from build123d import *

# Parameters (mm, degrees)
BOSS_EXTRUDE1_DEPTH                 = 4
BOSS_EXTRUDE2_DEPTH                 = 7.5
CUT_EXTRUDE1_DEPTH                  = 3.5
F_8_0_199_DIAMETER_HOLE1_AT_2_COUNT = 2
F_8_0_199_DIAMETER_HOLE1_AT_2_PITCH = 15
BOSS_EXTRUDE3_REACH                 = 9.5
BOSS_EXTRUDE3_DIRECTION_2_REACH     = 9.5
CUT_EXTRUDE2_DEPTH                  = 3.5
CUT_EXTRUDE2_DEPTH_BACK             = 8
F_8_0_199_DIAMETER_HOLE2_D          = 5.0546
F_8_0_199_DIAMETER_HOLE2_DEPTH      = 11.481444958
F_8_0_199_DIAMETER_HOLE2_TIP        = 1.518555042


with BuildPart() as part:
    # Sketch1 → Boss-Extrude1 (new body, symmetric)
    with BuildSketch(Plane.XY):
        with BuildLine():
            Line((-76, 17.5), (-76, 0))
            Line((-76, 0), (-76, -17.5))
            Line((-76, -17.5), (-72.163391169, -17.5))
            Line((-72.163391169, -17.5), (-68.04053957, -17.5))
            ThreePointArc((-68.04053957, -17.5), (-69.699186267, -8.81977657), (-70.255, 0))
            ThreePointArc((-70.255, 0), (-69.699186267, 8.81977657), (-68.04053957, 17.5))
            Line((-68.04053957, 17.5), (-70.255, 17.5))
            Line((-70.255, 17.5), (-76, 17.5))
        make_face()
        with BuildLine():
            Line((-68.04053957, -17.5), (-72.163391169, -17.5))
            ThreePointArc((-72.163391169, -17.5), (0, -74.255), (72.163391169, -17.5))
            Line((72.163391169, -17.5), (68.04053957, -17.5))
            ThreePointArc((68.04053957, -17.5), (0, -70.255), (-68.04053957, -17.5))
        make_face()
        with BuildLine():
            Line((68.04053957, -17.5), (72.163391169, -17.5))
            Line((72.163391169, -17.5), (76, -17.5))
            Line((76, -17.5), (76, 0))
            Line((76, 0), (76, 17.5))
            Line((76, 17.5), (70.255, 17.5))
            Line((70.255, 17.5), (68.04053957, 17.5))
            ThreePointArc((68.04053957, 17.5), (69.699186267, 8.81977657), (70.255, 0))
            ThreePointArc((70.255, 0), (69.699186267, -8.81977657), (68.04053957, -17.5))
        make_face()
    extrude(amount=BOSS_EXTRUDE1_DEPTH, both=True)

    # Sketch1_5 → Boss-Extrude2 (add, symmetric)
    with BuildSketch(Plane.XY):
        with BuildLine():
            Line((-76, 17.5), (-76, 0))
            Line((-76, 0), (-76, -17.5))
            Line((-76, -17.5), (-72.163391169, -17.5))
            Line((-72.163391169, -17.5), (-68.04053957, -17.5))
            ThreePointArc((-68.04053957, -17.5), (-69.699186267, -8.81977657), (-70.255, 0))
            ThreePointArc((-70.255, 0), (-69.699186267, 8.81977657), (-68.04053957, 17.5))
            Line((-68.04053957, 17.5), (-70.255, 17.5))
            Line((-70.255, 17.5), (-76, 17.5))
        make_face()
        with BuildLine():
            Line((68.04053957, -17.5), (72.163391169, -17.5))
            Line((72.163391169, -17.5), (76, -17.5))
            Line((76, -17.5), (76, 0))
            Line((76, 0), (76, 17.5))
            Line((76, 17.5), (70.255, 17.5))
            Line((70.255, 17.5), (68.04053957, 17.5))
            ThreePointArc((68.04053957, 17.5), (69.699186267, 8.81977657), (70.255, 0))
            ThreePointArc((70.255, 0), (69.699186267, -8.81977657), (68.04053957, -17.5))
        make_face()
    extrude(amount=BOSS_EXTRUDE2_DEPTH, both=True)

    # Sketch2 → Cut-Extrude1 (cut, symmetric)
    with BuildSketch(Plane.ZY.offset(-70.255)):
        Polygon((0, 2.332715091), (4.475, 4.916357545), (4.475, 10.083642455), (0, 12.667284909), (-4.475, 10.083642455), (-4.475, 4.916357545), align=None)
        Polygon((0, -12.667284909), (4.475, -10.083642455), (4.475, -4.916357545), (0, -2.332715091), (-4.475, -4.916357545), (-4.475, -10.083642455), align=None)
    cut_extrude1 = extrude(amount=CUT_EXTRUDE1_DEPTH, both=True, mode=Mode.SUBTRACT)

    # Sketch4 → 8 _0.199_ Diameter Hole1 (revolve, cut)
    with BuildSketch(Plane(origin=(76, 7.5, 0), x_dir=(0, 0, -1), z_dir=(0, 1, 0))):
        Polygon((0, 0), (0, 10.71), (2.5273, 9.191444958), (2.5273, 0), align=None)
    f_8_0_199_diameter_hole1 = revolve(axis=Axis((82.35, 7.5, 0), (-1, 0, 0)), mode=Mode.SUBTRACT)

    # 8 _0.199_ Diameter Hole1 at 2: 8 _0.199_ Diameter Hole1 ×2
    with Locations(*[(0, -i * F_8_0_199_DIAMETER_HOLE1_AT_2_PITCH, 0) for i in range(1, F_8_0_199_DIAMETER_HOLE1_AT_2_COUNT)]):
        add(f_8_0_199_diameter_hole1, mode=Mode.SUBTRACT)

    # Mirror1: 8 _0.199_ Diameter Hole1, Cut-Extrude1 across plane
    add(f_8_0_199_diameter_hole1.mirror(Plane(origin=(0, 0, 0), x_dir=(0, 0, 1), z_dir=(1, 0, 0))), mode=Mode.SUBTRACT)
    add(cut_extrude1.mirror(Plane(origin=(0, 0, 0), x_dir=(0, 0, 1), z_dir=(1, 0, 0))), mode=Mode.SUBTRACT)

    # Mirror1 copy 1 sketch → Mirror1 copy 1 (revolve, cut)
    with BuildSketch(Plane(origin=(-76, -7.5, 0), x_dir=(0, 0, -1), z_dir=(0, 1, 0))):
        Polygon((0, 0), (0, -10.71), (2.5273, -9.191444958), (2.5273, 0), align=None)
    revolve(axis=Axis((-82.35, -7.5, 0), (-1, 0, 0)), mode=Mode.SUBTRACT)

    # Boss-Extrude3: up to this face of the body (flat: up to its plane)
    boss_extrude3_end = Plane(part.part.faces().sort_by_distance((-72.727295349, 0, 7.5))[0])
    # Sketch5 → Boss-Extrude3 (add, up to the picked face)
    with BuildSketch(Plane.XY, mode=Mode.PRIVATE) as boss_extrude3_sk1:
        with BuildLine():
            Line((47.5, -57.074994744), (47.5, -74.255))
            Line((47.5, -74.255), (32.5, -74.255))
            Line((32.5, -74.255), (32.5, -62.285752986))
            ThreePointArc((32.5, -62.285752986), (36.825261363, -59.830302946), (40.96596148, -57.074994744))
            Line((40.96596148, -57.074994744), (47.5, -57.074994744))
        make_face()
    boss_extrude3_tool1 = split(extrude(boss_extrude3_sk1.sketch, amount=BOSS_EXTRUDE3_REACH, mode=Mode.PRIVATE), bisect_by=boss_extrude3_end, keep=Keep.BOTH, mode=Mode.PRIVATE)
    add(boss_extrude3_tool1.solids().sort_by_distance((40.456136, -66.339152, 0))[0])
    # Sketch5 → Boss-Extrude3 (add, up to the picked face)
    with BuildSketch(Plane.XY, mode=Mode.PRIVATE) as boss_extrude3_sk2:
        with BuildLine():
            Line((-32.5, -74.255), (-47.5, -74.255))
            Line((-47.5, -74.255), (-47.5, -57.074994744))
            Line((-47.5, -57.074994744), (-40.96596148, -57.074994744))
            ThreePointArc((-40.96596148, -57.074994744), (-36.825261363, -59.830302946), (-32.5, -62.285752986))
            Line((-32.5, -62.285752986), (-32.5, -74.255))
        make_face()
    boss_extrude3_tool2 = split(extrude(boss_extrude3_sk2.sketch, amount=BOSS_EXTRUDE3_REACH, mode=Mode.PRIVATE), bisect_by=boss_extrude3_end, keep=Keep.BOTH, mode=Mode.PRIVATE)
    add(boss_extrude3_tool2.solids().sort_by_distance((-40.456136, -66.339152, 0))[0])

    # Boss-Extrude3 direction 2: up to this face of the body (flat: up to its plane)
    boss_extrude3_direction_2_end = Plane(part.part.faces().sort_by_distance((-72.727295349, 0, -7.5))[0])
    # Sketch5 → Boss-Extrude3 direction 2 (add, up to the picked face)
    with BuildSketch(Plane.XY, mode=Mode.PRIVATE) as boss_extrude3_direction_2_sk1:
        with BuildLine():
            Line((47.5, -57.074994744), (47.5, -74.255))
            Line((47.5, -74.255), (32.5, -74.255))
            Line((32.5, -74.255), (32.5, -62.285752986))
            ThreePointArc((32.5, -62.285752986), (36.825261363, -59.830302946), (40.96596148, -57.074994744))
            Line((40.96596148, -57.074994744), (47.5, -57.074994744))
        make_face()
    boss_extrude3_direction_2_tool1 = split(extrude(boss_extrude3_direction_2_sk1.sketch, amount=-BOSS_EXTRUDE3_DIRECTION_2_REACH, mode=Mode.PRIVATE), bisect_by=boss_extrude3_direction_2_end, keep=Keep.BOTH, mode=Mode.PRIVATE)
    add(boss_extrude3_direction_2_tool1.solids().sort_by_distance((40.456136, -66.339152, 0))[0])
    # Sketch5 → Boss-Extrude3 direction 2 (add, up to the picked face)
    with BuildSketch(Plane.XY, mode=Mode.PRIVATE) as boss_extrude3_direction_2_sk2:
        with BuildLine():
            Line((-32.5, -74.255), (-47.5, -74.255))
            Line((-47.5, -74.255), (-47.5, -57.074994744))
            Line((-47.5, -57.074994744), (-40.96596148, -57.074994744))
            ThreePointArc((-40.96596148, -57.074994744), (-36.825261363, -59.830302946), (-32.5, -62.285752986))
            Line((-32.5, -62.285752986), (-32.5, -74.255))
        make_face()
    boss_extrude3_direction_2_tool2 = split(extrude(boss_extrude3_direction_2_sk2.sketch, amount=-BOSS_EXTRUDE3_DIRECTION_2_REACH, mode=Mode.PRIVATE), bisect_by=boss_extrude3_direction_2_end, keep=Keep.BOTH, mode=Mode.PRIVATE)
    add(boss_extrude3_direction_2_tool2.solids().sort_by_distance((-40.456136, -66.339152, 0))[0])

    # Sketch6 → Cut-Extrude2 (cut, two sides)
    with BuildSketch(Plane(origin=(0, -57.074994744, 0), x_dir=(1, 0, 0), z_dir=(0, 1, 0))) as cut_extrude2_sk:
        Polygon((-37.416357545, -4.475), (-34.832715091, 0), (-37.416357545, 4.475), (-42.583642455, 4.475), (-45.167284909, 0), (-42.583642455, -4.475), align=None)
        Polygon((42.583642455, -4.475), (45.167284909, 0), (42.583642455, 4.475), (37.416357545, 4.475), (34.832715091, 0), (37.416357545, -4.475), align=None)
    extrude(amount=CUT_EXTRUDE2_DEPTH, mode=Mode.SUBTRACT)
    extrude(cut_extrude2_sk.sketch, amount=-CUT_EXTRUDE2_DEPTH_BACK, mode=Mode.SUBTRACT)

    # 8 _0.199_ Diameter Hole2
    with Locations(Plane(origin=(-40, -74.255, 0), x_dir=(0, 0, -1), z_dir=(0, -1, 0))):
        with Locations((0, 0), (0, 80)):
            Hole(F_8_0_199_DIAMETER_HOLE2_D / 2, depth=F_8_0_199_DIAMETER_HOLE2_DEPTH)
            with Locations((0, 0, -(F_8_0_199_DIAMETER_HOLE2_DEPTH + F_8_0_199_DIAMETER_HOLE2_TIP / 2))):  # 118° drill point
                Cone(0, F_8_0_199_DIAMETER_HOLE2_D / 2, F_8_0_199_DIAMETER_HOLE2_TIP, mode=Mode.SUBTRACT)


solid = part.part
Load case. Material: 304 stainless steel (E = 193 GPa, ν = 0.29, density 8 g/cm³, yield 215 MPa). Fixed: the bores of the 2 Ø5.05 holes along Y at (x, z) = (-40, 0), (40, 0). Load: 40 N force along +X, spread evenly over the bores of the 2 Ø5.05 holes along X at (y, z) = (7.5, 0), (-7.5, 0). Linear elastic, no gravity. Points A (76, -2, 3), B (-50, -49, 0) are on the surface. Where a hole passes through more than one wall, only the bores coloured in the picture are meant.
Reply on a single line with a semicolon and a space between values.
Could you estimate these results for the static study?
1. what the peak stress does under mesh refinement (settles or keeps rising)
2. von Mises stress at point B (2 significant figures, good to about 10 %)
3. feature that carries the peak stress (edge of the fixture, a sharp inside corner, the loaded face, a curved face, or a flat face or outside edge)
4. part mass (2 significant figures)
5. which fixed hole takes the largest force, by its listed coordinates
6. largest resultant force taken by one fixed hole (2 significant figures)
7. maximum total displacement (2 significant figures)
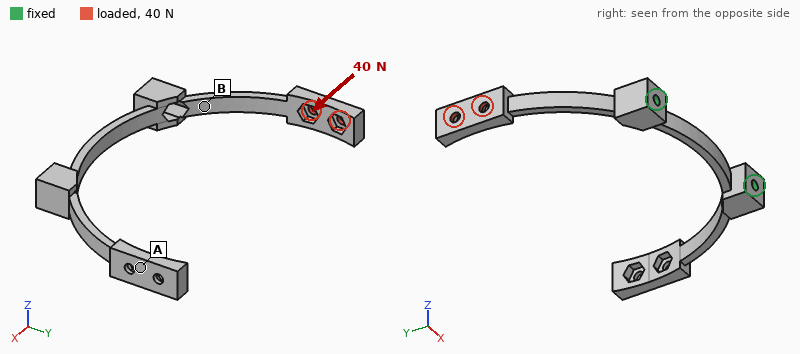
keeps rising; 97 MPa; a sharp inside corner; 130 g; (-40, 0); 40 N; 0.65 mm
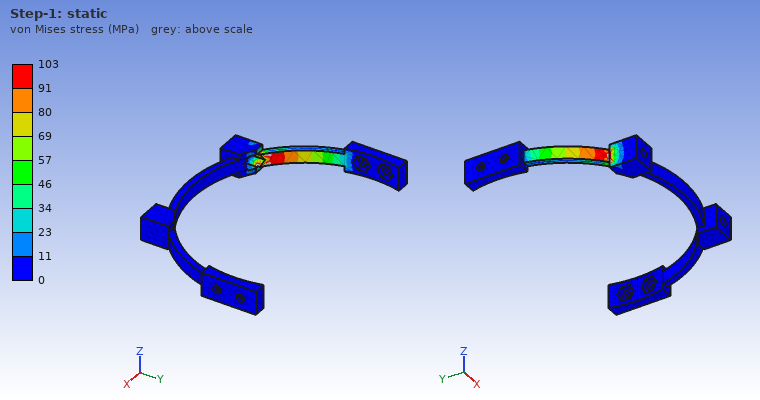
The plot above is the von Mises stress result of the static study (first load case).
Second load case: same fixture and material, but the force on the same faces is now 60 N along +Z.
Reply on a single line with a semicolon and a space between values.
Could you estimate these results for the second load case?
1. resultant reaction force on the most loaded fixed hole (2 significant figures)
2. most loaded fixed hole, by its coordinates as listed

62 N; (-40, 0)
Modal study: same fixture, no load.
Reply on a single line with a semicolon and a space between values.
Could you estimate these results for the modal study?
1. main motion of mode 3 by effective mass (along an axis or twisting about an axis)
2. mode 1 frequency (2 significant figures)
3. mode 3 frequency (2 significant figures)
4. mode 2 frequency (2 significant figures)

along Z; 290 Hz; 520 Hz; 290 Hz
